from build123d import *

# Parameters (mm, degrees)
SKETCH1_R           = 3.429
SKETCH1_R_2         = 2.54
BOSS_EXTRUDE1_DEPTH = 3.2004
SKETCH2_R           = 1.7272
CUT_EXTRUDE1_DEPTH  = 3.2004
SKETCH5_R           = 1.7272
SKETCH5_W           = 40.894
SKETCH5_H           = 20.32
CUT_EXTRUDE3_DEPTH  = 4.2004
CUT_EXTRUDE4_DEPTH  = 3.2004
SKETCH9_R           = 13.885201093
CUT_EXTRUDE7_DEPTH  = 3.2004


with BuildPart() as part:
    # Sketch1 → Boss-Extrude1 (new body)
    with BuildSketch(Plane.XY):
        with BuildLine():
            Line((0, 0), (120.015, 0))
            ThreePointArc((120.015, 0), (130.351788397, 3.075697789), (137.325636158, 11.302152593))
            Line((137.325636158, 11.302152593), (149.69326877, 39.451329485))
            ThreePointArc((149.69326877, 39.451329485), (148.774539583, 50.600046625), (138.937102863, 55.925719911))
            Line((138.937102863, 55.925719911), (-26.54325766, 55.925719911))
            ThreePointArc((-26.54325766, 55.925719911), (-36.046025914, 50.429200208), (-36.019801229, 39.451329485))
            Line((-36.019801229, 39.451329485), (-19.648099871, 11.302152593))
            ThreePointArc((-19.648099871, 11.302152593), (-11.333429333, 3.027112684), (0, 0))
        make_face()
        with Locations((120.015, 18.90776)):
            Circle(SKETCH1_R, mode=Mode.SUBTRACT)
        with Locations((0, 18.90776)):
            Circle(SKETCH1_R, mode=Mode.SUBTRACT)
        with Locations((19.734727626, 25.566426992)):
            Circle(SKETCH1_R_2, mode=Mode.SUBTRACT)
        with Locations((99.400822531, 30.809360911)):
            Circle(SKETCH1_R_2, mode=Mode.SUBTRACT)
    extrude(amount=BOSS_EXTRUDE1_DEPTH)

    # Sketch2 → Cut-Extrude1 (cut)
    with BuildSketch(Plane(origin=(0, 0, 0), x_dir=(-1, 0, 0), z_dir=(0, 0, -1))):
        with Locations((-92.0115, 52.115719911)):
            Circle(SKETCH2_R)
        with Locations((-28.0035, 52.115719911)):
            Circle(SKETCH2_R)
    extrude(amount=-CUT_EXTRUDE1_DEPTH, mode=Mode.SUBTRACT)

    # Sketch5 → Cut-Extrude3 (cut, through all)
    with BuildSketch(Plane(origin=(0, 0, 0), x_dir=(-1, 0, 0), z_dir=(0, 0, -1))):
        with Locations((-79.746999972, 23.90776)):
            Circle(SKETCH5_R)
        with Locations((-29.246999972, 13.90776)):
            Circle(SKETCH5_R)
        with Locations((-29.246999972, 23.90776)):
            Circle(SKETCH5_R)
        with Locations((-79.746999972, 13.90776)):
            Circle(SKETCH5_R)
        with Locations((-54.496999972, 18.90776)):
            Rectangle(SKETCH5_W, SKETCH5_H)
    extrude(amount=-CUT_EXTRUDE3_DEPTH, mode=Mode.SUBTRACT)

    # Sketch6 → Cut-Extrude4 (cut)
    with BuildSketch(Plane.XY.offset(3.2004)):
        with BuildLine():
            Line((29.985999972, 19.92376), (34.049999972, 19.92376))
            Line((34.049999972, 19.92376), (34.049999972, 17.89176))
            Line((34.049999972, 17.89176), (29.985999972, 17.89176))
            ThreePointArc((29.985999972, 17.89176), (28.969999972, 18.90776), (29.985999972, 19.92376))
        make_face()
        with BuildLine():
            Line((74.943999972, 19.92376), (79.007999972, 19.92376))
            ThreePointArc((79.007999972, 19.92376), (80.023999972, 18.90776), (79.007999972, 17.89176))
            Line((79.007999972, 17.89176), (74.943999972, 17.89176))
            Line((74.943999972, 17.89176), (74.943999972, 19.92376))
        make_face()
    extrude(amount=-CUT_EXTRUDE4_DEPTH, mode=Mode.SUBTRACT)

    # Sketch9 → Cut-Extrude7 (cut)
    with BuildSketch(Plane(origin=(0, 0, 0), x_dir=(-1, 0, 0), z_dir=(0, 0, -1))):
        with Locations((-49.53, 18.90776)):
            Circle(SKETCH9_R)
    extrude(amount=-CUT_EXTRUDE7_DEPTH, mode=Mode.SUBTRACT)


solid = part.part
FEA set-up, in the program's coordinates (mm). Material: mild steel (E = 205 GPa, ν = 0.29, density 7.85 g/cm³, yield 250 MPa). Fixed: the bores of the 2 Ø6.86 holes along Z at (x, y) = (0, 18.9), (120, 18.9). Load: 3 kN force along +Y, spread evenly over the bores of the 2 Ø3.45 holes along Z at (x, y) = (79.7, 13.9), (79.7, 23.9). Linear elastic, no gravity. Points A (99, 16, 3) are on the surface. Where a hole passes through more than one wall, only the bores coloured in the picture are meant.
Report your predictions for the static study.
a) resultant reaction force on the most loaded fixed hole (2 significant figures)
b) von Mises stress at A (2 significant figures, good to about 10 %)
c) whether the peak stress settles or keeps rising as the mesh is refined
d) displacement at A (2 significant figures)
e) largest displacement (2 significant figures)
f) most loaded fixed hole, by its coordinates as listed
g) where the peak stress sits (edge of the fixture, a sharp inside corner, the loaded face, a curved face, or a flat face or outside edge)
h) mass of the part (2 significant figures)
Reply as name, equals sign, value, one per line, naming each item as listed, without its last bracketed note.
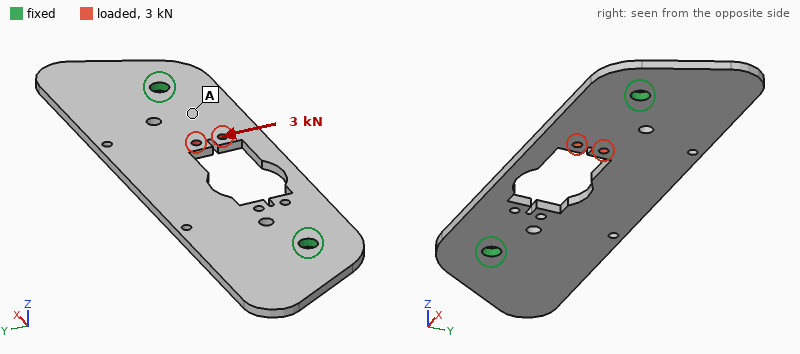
resultant reaction force on the most loaded fixed hole = 2.3 kN
von Mises stress at A = 19 MPa
whether the peak stress settles or keeps rising as the mesh is refined = keeps rising
displacement at A = 12 µm
largest displacement = 28 µm
most loaded fixed hole, by its coordinates as listed = (120, 18.9)
where the peak stress sits = edge of the fixture
mass of the part = 210 g
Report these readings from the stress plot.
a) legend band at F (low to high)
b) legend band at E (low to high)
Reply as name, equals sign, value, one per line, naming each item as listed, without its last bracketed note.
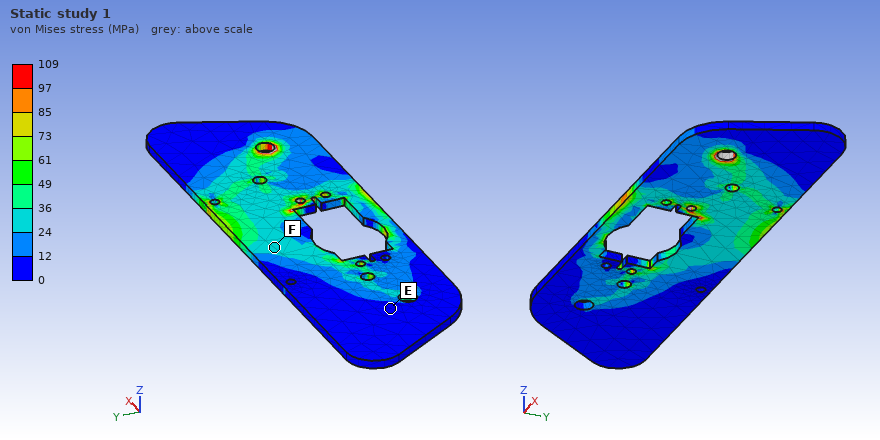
legend band at F = 24 to 36 MPa
legend band at E = 0 to 12 MPa
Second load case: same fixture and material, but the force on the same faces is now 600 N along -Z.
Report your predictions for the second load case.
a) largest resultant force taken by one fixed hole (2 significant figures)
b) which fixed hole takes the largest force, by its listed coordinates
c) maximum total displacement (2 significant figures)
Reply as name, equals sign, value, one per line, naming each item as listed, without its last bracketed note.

largest resultant force taken by one fixed hole = 450 N
which fixed hole takes the largest force, by its listed coordinates = (120, 18.9)
maximum total displacement = 0.23 mm
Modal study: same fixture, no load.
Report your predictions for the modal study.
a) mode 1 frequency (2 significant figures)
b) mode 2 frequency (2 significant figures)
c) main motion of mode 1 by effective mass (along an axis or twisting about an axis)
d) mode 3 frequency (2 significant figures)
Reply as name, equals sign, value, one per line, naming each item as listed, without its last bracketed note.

mode 1 frequency = 1000 Hz
mode 2 frequency = 1500 Hz
main motion of mode 1 by effective mass = along Z
mode 3 frequency = 1700 Hz
